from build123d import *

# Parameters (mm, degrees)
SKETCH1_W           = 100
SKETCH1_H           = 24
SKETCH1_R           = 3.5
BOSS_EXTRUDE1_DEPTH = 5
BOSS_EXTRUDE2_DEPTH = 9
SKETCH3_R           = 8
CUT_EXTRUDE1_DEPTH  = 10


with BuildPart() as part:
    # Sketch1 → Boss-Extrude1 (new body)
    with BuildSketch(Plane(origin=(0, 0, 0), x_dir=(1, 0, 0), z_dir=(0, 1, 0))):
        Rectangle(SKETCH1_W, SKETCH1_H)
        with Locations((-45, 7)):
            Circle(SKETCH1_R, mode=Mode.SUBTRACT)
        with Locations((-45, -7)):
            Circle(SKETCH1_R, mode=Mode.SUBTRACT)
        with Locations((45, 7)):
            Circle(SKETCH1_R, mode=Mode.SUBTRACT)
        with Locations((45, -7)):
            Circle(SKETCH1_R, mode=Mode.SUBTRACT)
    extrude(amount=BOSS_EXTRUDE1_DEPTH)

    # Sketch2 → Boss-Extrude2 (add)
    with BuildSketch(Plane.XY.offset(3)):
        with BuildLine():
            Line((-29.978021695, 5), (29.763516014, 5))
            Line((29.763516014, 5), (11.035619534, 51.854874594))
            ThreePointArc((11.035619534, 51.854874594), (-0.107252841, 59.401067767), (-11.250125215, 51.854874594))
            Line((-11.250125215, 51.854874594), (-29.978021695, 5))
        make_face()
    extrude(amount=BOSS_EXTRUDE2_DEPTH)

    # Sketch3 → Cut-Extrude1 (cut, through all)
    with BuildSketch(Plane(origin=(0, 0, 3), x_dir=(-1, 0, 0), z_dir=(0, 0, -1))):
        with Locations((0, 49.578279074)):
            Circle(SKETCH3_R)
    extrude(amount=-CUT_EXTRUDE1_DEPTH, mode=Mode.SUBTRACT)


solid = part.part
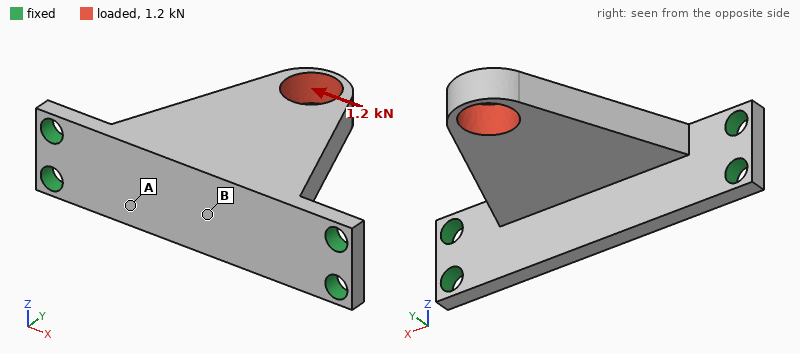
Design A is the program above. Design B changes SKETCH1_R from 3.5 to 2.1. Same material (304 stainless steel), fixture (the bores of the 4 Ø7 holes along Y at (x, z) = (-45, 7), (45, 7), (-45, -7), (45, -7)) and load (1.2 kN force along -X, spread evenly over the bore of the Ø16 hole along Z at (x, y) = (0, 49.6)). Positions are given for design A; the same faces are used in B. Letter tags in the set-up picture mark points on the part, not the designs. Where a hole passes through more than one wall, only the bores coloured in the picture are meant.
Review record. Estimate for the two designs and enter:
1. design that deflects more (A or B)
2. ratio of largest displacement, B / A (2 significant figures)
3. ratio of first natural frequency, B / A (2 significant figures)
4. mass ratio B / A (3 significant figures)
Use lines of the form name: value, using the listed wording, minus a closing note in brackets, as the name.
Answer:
design that deflects more: B
ratio of largest displacement, B / A: 1.1
ratio of first natural frequency, B / A: 0.95
mass ratio B / A: 1.02
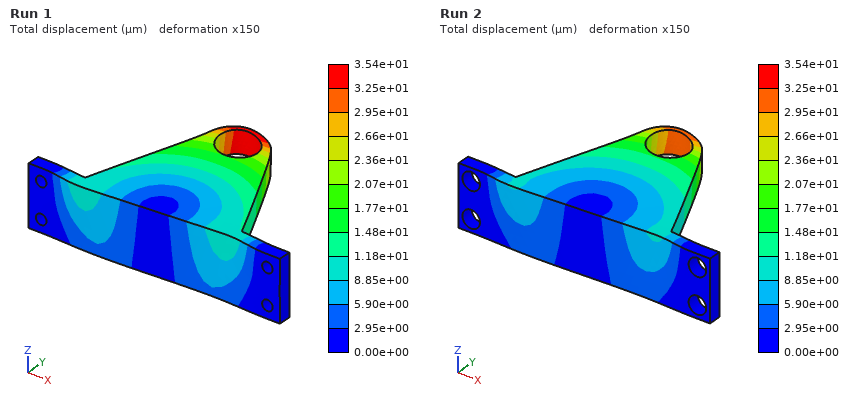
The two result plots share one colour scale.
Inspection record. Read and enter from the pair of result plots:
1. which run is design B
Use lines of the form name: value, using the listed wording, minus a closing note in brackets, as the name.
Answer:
which run is design B: Run 1
